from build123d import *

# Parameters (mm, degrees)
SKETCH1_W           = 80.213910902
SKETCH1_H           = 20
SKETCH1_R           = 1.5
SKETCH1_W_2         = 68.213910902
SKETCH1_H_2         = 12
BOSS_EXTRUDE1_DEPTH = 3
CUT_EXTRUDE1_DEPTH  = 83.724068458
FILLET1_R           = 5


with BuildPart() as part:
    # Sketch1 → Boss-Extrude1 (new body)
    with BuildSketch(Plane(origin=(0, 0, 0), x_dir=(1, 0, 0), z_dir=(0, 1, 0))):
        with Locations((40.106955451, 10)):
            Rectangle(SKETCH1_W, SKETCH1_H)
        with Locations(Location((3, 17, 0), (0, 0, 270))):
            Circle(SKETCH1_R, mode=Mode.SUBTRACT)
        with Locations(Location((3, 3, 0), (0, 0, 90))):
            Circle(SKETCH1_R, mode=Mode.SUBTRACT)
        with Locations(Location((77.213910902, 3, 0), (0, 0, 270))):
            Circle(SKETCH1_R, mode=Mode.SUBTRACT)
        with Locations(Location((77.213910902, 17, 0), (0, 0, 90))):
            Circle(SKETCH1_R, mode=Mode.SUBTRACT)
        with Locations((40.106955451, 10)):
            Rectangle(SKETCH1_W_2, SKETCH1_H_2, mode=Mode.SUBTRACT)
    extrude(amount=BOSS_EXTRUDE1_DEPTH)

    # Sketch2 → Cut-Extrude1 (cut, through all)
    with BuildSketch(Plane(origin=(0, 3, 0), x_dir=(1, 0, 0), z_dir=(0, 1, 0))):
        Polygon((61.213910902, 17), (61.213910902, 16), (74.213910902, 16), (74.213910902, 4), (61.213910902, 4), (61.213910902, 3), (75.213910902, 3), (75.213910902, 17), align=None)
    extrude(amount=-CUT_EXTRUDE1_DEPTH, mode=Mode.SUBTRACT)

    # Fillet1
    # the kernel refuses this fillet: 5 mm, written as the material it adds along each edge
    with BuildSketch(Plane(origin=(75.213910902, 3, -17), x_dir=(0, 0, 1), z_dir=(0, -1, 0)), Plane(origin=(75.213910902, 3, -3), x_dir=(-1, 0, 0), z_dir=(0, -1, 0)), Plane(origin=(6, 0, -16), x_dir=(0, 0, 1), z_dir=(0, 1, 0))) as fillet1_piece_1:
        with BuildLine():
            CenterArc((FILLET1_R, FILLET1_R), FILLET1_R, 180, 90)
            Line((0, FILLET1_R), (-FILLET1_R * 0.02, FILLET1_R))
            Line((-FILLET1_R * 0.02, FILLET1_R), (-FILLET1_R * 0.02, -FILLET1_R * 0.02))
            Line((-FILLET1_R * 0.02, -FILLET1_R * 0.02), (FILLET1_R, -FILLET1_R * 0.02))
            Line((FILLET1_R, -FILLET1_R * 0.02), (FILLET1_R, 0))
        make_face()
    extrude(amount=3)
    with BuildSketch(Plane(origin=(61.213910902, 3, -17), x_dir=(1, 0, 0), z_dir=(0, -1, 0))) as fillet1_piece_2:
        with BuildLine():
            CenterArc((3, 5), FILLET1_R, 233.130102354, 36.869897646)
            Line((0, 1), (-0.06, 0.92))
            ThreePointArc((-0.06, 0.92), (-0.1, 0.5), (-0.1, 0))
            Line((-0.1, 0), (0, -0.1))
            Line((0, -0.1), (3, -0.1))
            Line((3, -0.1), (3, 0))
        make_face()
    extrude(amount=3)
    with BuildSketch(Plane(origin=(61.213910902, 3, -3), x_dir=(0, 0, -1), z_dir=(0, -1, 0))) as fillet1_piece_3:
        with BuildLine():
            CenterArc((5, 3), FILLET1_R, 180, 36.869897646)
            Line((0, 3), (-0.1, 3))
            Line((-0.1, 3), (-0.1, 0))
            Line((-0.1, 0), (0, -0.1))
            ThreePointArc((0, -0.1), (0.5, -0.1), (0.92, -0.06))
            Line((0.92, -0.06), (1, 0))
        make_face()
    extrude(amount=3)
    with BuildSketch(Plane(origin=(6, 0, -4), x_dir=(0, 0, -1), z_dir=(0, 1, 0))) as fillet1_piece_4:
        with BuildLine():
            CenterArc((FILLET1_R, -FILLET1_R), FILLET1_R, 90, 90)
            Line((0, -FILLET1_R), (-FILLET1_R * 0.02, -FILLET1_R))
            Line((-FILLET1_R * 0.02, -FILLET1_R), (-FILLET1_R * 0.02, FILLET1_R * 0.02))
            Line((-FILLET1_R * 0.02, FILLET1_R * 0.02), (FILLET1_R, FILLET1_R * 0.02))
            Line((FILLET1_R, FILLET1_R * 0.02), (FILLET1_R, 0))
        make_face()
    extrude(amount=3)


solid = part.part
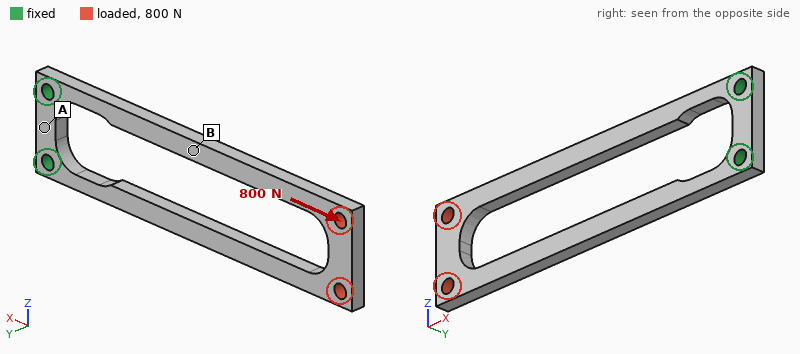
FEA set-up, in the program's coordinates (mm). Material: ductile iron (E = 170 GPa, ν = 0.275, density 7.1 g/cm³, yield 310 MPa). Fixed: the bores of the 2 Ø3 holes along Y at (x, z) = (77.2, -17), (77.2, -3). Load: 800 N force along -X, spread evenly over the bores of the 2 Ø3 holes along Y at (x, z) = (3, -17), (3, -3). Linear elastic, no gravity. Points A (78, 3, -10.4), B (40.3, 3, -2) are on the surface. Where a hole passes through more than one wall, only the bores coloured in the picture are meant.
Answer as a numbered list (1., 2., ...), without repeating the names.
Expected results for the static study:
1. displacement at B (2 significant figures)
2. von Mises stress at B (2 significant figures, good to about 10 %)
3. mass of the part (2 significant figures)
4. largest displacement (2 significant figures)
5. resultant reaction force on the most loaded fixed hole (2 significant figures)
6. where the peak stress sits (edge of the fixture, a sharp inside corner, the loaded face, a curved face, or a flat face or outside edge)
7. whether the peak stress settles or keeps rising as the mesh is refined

1. 8.3 µm
2. 33 MPa
3. 16 g
4. 17 µm
5. 400 N
6. edge of the fixture
7. keeps rising
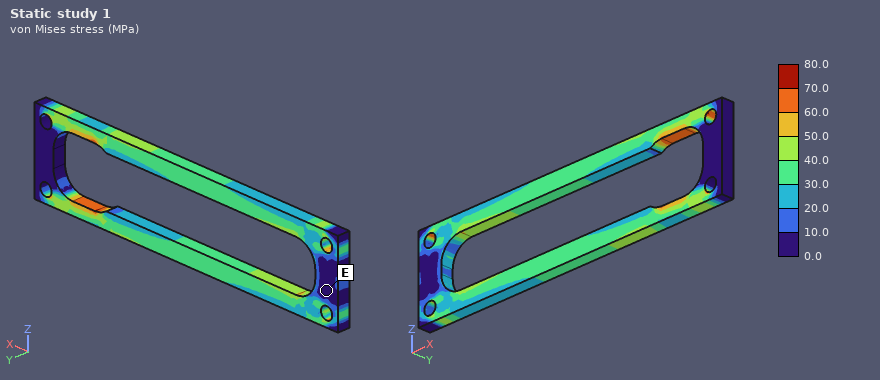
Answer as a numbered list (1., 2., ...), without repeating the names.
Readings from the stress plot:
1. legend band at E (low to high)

1. 0.0 to 10.0 MPa
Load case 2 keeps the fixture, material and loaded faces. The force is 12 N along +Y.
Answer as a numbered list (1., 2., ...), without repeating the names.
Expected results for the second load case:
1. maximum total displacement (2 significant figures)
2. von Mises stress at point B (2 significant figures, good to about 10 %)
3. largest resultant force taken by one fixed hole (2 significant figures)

1. 0.60 mm
2. 37 MPa
3. 6.0 N
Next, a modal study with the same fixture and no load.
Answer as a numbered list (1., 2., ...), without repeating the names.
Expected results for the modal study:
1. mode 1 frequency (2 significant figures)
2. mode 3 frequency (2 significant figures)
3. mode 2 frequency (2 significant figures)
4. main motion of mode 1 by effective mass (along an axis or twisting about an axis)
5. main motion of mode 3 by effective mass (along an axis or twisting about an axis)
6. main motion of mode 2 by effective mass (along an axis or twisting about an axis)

1. 330 Hz
2. 1600 Hz
3. 730 Hz
4. along Y
5. twisting about X
6. along Z
